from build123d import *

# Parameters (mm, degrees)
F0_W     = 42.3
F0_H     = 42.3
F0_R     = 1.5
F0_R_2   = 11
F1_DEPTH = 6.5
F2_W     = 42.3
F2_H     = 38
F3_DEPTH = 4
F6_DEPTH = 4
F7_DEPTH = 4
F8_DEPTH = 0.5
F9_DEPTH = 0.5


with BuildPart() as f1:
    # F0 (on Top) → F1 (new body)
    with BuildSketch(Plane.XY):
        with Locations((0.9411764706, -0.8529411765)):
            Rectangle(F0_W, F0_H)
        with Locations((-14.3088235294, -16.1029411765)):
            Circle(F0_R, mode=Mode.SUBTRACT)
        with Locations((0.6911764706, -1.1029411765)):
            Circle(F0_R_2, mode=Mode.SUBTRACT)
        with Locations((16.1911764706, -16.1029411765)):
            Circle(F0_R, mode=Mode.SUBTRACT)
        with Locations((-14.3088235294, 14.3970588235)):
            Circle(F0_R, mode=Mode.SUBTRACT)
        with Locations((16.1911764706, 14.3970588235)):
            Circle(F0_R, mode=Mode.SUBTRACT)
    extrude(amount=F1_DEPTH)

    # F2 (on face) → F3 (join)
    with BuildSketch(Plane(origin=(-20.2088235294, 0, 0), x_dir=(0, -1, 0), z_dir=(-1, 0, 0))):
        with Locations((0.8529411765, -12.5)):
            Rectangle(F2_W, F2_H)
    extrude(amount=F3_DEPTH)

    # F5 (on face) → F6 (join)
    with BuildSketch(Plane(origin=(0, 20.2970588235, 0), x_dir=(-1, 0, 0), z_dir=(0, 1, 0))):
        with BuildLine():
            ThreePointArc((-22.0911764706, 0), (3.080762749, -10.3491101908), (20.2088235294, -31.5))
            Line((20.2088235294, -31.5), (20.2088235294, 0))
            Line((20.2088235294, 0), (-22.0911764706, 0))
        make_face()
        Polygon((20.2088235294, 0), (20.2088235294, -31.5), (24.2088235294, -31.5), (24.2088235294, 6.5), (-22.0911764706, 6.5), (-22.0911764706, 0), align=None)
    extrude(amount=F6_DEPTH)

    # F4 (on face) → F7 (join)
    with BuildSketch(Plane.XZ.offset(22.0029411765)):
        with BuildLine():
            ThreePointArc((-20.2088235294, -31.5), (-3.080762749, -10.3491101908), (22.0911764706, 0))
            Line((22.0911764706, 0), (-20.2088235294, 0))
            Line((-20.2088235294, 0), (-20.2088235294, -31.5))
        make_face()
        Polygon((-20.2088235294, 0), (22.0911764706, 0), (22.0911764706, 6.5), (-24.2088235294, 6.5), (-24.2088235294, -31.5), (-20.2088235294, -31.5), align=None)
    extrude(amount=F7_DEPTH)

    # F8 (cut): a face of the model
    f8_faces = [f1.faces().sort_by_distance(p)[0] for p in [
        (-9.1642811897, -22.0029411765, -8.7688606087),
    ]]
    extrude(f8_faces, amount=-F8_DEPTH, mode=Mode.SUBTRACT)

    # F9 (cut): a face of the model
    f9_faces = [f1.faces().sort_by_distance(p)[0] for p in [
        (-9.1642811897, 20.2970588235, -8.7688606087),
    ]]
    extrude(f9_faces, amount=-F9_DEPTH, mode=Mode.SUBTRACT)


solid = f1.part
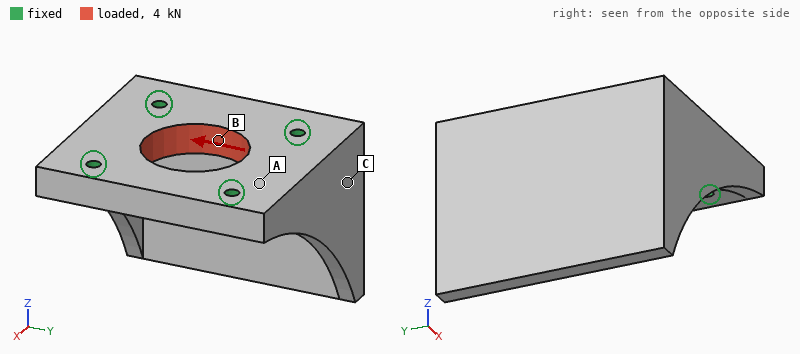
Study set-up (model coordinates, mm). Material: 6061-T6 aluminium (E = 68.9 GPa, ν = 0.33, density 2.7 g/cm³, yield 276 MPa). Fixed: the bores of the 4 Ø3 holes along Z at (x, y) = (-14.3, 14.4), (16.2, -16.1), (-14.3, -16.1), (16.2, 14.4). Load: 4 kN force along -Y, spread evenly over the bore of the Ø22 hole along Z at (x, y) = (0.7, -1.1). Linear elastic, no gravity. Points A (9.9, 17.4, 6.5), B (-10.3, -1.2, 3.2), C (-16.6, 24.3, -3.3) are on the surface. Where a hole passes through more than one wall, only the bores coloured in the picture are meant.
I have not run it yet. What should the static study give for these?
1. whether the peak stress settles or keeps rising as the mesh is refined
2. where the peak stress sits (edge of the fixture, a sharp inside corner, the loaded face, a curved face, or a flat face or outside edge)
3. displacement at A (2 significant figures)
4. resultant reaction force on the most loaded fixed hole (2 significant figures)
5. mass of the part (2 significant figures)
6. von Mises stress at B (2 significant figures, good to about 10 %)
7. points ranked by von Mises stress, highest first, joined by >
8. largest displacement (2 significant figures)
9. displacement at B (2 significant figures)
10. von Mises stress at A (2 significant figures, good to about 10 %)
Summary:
keeps rising
edge of the fixture
2.0 µm
1.0 kN
59 g
15 MPa
B > A > C
4.2 µm
2.3 µm
8.2 MPa
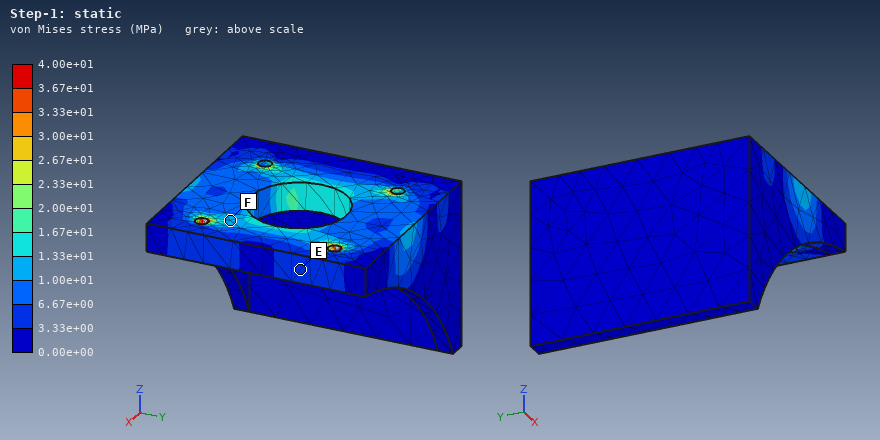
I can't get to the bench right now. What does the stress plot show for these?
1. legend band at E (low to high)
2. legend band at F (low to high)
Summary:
3.33e+00 to 6.67e+00 MPa
1.00e+01 to 1.33e+01 MPa
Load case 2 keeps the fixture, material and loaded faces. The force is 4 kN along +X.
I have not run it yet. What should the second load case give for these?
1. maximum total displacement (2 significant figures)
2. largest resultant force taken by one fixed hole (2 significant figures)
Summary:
5.5 µm
1.0 kN
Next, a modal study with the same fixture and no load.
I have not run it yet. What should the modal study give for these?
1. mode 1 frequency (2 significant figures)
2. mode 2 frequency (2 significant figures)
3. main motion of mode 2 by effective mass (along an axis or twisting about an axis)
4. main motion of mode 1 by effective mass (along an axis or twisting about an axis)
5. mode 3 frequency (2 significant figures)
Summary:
5700 Hz
8500 Hz
along Y
along X
13 kHz
